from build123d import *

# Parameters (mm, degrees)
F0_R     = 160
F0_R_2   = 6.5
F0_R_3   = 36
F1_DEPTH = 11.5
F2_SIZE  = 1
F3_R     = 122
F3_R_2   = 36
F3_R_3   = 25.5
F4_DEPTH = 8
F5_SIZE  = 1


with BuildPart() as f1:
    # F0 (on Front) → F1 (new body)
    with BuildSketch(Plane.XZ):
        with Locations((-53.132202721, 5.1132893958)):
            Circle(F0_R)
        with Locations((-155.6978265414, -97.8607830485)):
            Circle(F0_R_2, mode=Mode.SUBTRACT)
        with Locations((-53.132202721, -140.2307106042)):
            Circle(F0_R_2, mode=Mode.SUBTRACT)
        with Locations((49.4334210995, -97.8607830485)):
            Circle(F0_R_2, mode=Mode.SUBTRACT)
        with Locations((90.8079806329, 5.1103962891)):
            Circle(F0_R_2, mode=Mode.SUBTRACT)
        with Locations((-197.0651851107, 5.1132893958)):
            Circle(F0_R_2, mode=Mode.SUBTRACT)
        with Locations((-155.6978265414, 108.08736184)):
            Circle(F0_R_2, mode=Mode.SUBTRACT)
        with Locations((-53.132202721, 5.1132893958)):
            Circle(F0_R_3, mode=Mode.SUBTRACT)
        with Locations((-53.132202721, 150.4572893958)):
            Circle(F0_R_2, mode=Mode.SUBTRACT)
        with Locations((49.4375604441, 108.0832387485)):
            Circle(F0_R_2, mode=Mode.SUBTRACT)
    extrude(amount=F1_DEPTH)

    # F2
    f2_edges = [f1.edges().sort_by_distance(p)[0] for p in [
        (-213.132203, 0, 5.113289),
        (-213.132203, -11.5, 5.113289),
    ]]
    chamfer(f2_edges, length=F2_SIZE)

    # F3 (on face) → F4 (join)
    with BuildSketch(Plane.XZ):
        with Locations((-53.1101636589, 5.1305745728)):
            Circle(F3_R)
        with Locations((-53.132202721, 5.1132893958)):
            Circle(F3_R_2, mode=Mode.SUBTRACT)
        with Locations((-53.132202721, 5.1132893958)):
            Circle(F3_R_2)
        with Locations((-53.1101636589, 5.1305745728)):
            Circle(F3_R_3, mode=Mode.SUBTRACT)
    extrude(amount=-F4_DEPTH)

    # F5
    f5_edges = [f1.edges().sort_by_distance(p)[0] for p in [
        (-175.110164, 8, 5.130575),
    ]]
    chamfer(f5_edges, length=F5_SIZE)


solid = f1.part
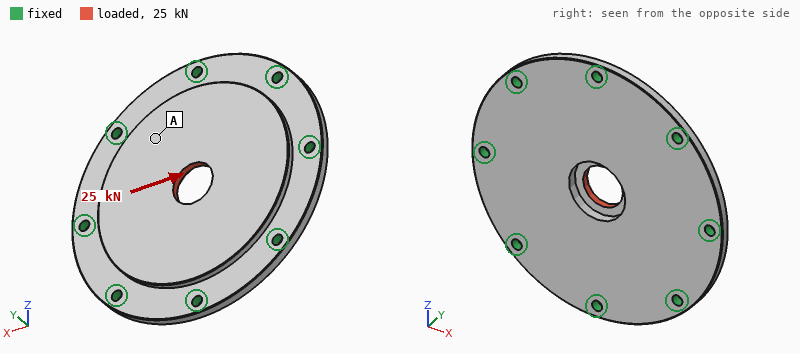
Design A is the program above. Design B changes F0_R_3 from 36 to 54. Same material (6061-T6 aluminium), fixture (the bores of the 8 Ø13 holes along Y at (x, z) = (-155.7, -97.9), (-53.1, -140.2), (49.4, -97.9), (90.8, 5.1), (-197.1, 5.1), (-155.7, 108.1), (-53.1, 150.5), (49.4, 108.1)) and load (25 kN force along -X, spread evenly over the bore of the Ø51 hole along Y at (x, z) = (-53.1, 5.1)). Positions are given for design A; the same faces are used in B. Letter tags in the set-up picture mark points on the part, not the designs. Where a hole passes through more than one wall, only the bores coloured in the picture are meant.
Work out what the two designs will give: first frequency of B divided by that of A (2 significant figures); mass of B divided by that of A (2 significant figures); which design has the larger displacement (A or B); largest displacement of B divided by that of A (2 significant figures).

1.1
0.95
B
1.3
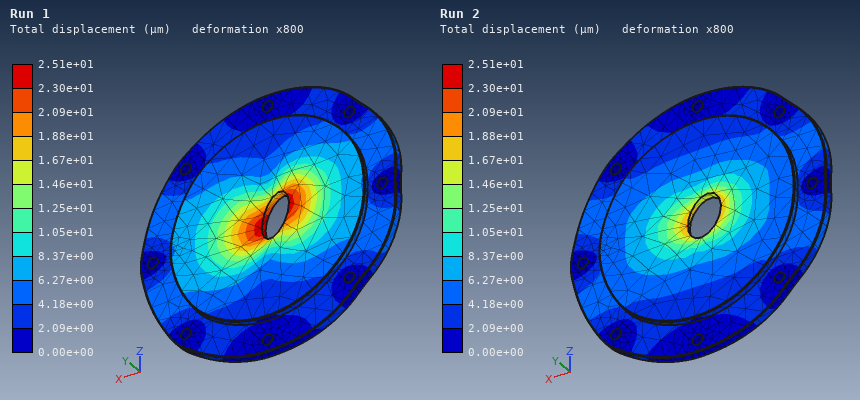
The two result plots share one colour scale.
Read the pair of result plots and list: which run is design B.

Run 1
